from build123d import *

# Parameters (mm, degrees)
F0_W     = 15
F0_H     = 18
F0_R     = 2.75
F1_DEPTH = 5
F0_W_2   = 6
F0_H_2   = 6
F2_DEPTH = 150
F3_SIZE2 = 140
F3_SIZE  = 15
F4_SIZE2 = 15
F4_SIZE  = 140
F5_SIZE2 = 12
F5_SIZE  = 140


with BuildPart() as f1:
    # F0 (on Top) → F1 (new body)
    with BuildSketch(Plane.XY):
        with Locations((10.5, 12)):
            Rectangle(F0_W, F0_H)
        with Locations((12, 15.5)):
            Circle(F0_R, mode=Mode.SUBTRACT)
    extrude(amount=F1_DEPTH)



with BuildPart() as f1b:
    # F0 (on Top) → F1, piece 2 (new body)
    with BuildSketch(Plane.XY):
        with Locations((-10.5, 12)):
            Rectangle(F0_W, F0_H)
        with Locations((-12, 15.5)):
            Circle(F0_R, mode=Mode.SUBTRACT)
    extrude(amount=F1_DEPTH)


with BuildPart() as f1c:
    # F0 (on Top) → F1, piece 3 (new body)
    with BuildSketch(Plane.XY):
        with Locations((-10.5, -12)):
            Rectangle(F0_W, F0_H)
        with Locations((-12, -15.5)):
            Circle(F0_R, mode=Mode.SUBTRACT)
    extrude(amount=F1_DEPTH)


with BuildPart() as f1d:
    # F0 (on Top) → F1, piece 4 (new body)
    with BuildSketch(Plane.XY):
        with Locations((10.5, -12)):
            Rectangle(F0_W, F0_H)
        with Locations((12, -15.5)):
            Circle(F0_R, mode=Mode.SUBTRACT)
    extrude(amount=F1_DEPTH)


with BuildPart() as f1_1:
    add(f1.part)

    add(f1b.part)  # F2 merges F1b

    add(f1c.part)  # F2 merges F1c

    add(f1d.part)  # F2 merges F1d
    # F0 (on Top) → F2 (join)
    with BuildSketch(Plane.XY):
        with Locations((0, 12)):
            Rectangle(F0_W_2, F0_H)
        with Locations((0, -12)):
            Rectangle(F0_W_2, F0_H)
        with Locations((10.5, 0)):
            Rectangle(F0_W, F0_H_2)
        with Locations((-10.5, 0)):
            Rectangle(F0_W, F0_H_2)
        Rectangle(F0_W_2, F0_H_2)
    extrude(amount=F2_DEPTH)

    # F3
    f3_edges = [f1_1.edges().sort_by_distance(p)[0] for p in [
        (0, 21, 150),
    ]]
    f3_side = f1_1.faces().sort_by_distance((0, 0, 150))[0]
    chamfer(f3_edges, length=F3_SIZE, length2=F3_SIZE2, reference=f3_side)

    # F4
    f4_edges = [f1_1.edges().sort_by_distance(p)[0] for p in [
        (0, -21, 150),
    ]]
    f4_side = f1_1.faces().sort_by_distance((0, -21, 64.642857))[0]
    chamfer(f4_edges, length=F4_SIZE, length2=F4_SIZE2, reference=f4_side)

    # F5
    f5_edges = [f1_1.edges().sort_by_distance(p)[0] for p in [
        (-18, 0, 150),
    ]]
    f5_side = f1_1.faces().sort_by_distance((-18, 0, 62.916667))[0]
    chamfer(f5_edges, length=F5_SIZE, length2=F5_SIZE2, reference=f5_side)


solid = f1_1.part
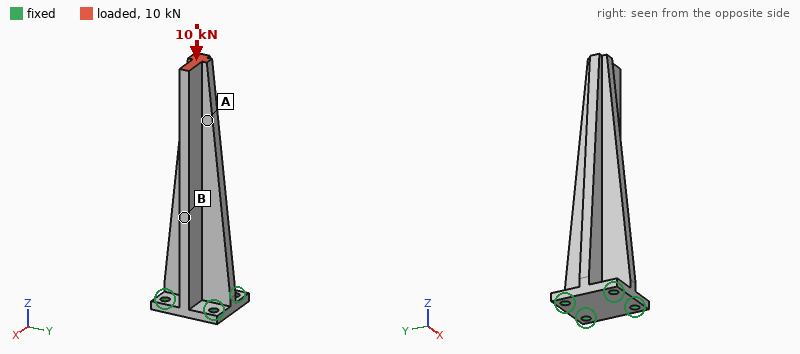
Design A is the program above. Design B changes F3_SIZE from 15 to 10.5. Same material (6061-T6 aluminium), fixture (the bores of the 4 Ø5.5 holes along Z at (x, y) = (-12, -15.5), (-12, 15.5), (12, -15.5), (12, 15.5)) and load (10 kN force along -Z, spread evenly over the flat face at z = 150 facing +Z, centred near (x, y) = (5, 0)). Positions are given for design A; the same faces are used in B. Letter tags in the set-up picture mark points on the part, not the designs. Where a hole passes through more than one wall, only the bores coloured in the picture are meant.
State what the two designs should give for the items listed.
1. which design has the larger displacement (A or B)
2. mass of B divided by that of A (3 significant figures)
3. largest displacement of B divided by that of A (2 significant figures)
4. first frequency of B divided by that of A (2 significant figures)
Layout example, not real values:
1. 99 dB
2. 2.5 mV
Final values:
1. A
2. 1.04
3. 0.87
4. 0.96
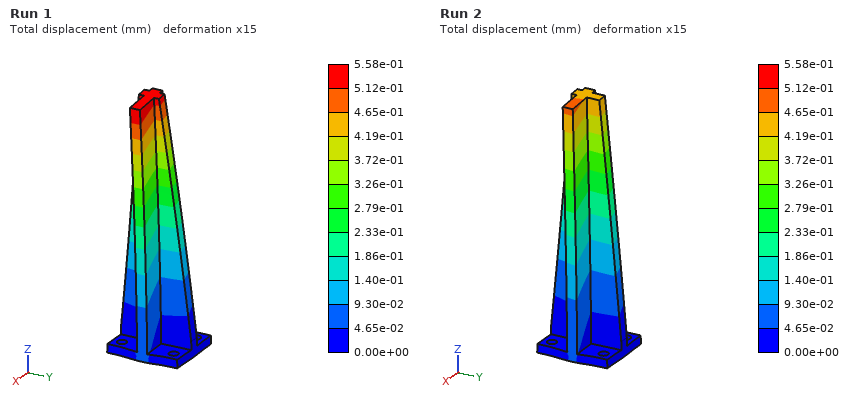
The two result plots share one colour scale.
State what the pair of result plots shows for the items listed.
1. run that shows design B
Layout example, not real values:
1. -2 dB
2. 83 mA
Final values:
1. Run 2
